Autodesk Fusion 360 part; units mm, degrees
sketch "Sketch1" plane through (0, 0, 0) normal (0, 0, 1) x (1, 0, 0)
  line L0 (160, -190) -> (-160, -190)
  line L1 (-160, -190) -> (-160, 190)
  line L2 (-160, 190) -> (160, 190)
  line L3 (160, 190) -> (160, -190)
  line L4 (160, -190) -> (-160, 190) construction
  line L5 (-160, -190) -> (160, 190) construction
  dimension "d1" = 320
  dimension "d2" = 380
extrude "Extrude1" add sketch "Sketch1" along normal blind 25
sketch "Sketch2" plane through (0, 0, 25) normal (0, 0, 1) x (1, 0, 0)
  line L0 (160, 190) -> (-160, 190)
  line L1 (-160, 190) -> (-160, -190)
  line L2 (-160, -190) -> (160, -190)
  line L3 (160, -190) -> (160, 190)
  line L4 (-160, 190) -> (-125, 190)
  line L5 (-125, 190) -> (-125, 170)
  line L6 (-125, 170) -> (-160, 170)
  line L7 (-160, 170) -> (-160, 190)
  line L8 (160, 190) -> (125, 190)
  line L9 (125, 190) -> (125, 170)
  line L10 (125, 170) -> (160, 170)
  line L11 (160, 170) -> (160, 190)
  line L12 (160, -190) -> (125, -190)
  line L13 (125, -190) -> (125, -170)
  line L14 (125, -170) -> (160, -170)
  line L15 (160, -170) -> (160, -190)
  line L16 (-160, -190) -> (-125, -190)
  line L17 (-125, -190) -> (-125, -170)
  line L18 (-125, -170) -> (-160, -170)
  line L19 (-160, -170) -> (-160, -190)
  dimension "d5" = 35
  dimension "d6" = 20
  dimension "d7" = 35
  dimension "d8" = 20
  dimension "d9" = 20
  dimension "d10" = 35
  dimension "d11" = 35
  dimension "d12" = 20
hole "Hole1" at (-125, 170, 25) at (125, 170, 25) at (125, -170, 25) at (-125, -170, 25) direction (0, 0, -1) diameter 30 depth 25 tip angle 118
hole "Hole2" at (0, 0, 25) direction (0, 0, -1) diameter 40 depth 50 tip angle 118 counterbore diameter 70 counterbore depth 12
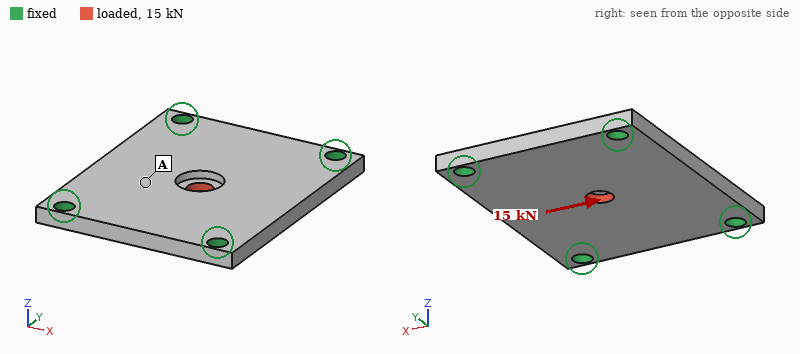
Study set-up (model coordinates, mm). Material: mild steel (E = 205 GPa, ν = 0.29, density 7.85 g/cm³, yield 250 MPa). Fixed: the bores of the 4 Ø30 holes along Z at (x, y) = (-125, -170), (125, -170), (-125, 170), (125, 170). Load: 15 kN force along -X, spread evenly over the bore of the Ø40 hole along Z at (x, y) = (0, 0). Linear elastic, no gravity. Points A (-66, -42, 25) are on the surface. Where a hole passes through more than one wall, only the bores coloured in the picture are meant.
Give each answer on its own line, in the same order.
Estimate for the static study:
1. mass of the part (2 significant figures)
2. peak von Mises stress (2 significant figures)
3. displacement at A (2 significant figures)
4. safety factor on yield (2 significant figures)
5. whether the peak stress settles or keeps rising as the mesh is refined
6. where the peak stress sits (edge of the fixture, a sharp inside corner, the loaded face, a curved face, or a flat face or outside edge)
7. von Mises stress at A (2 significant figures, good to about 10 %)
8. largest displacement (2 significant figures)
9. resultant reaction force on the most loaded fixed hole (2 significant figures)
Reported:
23 kg
16 MPa
2.3 µm
15
settles
the loaded face
1.5 MPa
4.1 µm
4.5 kN
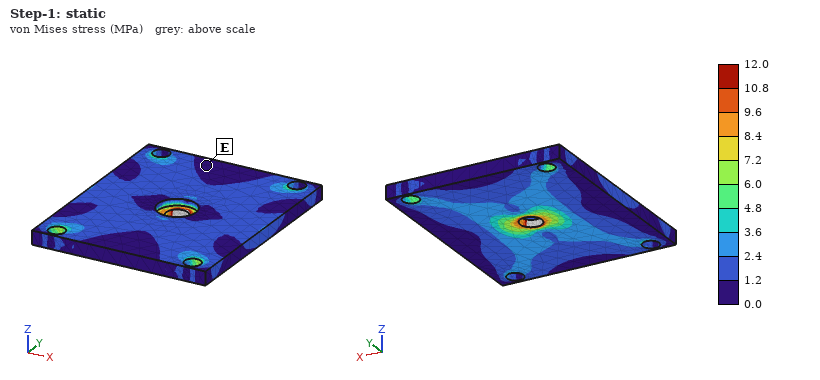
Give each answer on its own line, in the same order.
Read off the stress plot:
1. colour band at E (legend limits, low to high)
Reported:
0.0 to 1.2 MPa
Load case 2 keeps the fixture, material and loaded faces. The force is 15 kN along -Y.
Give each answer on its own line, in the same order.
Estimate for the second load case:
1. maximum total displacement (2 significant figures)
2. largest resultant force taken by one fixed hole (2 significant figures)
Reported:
3.3 µm
4.1 kN
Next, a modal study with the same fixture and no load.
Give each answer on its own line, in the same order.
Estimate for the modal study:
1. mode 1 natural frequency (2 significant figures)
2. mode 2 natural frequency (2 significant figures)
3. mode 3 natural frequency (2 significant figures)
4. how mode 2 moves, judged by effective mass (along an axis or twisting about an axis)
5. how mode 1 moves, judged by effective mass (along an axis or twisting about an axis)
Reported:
950 Hz
1400 Hz
1900 Hz
twisting about Y
along Z
